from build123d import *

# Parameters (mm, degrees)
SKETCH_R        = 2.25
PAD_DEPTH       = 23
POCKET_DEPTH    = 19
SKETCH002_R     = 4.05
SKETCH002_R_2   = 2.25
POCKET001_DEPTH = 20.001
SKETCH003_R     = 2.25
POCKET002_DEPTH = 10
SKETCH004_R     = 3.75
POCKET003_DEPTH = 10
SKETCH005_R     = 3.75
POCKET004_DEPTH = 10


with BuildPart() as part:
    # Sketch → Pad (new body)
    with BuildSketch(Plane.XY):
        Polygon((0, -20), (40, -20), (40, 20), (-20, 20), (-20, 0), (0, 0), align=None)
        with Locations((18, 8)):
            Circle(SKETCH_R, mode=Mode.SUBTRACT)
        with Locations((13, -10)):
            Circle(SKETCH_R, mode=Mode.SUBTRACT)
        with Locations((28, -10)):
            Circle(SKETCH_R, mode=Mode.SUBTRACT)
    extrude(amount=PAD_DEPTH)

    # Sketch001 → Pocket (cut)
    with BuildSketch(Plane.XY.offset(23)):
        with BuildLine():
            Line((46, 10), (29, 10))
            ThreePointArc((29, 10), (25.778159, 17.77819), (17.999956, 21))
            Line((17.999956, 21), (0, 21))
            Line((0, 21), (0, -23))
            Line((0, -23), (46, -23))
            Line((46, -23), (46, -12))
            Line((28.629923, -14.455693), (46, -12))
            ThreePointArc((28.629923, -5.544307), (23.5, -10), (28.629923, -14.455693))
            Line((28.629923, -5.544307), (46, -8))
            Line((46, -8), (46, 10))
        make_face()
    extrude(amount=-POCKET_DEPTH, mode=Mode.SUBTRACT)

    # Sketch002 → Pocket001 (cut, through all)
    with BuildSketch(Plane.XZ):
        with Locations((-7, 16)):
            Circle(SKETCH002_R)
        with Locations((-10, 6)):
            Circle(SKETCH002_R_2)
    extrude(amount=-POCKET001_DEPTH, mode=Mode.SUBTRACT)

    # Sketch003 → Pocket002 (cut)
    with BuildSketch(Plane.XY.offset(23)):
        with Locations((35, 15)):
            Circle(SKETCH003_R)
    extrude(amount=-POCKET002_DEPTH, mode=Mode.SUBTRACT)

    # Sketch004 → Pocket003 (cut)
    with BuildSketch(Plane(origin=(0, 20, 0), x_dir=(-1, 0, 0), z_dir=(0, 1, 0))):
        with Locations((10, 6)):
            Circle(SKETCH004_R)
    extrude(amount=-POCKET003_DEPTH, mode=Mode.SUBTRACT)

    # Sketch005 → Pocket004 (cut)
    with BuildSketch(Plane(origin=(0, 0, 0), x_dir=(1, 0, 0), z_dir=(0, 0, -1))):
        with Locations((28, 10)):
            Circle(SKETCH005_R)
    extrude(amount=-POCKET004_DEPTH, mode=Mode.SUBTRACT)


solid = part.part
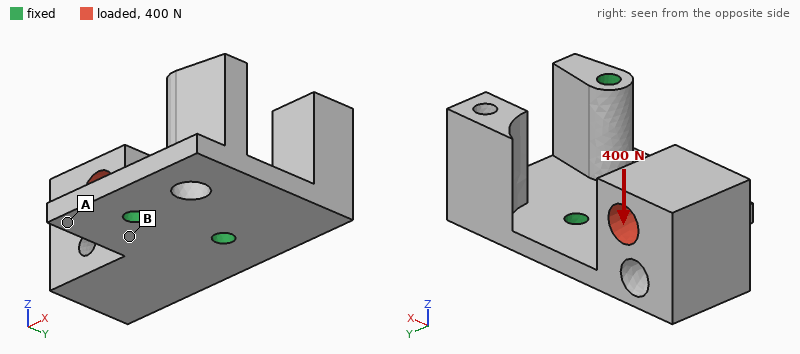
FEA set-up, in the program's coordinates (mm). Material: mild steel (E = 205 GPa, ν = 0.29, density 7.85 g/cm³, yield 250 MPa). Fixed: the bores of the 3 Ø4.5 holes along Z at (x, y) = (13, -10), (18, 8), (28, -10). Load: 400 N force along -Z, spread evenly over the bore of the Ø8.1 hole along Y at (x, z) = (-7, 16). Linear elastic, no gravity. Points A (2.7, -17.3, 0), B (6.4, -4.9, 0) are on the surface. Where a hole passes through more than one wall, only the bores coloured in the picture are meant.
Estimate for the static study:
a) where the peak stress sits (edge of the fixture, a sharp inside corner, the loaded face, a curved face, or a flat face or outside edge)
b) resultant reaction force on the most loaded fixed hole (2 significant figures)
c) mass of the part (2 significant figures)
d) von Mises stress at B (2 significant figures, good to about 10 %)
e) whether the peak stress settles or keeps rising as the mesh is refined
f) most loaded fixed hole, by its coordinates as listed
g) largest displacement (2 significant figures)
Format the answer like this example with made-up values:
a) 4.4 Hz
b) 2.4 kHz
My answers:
a) edge of the fixture
b) 310 N
c) 140 g
d) 65 MPa
e) keeps rising
f) (18, 8)
g) 0.13 mm
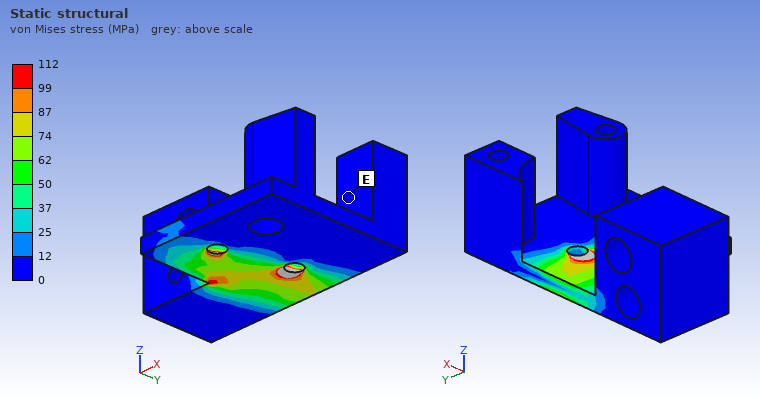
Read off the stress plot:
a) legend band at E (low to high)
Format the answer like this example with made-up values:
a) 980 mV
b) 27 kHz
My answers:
a) 0 to 12 MPa
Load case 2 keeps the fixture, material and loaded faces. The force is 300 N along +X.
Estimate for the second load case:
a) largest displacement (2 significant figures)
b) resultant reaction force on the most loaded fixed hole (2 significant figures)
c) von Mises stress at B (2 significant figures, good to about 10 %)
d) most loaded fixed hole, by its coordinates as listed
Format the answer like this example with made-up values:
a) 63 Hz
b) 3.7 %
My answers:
a) 93 µm
b) 310 N
c) 39 MPa
d) (18, 8)
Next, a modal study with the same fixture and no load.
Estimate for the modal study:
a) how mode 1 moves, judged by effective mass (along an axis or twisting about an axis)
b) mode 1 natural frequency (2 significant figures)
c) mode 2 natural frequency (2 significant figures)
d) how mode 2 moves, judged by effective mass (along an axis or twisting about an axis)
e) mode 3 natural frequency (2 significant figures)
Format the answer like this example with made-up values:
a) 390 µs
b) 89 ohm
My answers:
a) along Z
b) 1200 Hz
c) 3000 Hz
d) along Y
e) 3400 Hz
